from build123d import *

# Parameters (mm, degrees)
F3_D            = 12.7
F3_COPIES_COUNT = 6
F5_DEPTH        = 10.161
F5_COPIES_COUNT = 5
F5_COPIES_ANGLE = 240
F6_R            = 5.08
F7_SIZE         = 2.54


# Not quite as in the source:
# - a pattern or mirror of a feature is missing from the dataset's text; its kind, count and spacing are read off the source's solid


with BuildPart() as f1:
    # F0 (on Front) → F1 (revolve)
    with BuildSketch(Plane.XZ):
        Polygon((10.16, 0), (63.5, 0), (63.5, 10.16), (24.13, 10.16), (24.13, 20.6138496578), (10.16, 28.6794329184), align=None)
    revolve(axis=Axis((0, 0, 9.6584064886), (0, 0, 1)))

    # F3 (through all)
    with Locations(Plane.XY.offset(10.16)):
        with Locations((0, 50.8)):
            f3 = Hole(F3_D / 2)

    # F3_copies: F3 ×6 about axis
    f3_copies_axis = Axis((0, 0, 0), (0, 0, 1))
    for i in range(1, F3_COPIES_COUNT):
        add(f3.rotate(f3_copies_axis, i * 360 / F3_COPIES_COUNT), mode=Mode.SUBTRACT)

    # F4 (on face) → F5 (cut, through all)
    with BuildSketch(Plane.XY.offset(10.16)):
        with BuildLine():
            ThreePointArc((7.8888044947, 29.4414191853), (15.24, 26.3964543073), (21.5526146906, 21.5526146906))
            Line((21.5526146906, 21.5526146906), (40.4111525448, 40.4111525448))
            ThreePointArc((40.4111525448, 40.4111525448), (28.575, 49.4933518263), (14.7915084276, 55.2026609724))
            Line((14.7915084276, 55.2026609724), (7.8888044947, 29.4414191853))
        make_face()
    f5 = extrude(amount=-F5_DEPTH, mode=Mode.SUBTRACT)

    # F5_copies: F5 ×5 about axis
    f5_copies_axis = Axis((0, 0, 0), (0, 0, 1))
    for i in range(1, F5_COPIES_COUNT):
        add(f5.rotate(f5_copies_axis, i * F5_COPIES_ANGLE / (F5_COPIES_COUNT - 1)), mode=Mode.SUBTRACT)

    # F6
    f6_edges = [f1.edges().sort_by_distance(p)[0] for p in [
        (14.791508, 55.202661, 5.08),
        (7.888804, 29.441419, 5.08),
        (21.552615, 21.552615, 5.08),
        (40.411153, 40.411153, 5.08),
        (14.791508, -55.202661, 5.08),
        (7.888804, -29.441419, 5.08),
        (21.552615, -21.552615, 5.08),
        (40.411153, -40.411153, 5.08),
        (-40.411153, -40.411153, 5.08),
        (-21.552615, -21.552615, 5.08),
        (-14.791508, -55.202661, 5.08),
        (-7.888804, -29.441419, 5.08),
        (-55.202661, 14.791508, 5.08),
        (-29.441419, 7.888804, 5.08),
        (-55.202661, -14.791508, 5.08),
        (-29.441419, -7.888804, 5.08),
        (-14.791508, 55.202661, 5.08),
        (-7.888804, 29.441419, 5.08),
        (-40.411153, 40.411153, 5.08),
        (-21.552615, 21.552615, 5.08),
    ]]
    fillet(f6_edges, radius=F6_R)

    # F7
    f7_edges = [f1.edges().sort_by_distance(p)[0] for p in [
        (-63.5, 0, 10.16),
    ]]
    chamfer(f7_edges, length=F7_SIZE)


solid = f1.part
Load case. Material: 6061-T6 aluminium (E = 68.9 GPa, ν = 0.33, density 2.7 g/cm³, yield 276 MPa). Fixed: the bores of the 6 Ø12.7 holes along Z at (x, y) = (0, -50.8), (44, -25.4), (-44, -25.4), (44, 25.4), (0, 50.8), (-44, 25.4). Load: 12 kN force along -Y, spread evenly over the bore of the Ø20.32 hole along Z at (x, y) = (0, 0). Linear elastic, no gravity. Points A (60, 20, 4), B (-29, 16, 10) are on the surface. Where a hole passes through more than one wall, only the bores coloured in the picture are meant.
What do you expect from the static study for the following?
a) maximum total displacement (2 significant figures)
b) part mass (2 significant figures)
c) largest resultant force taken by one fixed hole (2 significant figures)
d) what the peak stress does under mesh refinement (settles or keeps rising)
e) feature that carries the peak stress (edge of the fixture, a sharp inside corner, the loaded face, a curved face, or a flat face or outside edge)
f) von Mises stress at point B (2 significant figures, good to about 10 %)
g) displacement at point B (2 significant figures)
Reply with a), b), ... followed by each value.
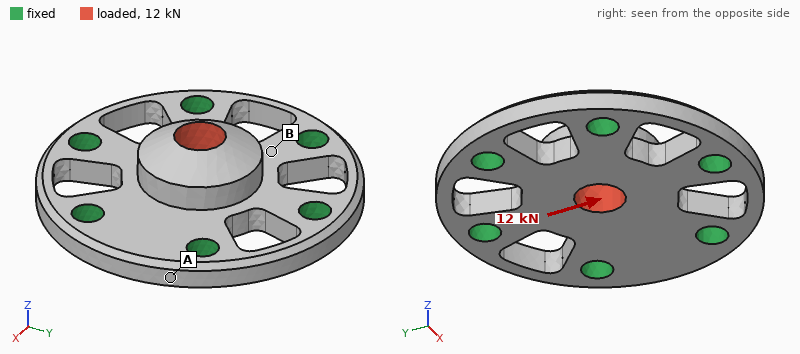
a) 22 µm
b) 290 g
c) 3.4 kN
d) keeps rising
e) edge of the fixture
f) 17 MPa
g) 4.4 µm
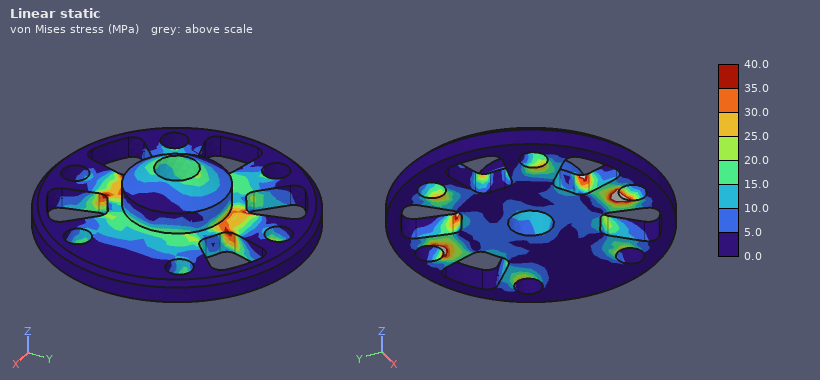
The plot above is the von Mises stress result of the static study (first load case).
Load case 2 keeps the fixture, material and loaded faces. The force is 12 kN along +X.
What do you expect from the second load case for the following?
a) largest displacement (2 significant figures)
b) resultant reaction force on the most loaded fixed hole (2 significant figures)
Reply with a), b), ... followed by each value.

a) 21 µm
b) 3.1 kN
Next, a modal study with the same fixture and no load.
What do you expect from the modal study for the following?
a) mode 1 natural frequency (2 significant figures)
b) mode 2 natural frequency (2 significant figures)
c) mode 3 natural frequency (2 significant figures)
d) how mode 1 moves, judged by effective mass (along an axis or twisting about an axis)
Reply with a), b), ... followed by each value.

a) 8500 Hz
b) 13 kHz
c) 13 kHz
d) along Z
